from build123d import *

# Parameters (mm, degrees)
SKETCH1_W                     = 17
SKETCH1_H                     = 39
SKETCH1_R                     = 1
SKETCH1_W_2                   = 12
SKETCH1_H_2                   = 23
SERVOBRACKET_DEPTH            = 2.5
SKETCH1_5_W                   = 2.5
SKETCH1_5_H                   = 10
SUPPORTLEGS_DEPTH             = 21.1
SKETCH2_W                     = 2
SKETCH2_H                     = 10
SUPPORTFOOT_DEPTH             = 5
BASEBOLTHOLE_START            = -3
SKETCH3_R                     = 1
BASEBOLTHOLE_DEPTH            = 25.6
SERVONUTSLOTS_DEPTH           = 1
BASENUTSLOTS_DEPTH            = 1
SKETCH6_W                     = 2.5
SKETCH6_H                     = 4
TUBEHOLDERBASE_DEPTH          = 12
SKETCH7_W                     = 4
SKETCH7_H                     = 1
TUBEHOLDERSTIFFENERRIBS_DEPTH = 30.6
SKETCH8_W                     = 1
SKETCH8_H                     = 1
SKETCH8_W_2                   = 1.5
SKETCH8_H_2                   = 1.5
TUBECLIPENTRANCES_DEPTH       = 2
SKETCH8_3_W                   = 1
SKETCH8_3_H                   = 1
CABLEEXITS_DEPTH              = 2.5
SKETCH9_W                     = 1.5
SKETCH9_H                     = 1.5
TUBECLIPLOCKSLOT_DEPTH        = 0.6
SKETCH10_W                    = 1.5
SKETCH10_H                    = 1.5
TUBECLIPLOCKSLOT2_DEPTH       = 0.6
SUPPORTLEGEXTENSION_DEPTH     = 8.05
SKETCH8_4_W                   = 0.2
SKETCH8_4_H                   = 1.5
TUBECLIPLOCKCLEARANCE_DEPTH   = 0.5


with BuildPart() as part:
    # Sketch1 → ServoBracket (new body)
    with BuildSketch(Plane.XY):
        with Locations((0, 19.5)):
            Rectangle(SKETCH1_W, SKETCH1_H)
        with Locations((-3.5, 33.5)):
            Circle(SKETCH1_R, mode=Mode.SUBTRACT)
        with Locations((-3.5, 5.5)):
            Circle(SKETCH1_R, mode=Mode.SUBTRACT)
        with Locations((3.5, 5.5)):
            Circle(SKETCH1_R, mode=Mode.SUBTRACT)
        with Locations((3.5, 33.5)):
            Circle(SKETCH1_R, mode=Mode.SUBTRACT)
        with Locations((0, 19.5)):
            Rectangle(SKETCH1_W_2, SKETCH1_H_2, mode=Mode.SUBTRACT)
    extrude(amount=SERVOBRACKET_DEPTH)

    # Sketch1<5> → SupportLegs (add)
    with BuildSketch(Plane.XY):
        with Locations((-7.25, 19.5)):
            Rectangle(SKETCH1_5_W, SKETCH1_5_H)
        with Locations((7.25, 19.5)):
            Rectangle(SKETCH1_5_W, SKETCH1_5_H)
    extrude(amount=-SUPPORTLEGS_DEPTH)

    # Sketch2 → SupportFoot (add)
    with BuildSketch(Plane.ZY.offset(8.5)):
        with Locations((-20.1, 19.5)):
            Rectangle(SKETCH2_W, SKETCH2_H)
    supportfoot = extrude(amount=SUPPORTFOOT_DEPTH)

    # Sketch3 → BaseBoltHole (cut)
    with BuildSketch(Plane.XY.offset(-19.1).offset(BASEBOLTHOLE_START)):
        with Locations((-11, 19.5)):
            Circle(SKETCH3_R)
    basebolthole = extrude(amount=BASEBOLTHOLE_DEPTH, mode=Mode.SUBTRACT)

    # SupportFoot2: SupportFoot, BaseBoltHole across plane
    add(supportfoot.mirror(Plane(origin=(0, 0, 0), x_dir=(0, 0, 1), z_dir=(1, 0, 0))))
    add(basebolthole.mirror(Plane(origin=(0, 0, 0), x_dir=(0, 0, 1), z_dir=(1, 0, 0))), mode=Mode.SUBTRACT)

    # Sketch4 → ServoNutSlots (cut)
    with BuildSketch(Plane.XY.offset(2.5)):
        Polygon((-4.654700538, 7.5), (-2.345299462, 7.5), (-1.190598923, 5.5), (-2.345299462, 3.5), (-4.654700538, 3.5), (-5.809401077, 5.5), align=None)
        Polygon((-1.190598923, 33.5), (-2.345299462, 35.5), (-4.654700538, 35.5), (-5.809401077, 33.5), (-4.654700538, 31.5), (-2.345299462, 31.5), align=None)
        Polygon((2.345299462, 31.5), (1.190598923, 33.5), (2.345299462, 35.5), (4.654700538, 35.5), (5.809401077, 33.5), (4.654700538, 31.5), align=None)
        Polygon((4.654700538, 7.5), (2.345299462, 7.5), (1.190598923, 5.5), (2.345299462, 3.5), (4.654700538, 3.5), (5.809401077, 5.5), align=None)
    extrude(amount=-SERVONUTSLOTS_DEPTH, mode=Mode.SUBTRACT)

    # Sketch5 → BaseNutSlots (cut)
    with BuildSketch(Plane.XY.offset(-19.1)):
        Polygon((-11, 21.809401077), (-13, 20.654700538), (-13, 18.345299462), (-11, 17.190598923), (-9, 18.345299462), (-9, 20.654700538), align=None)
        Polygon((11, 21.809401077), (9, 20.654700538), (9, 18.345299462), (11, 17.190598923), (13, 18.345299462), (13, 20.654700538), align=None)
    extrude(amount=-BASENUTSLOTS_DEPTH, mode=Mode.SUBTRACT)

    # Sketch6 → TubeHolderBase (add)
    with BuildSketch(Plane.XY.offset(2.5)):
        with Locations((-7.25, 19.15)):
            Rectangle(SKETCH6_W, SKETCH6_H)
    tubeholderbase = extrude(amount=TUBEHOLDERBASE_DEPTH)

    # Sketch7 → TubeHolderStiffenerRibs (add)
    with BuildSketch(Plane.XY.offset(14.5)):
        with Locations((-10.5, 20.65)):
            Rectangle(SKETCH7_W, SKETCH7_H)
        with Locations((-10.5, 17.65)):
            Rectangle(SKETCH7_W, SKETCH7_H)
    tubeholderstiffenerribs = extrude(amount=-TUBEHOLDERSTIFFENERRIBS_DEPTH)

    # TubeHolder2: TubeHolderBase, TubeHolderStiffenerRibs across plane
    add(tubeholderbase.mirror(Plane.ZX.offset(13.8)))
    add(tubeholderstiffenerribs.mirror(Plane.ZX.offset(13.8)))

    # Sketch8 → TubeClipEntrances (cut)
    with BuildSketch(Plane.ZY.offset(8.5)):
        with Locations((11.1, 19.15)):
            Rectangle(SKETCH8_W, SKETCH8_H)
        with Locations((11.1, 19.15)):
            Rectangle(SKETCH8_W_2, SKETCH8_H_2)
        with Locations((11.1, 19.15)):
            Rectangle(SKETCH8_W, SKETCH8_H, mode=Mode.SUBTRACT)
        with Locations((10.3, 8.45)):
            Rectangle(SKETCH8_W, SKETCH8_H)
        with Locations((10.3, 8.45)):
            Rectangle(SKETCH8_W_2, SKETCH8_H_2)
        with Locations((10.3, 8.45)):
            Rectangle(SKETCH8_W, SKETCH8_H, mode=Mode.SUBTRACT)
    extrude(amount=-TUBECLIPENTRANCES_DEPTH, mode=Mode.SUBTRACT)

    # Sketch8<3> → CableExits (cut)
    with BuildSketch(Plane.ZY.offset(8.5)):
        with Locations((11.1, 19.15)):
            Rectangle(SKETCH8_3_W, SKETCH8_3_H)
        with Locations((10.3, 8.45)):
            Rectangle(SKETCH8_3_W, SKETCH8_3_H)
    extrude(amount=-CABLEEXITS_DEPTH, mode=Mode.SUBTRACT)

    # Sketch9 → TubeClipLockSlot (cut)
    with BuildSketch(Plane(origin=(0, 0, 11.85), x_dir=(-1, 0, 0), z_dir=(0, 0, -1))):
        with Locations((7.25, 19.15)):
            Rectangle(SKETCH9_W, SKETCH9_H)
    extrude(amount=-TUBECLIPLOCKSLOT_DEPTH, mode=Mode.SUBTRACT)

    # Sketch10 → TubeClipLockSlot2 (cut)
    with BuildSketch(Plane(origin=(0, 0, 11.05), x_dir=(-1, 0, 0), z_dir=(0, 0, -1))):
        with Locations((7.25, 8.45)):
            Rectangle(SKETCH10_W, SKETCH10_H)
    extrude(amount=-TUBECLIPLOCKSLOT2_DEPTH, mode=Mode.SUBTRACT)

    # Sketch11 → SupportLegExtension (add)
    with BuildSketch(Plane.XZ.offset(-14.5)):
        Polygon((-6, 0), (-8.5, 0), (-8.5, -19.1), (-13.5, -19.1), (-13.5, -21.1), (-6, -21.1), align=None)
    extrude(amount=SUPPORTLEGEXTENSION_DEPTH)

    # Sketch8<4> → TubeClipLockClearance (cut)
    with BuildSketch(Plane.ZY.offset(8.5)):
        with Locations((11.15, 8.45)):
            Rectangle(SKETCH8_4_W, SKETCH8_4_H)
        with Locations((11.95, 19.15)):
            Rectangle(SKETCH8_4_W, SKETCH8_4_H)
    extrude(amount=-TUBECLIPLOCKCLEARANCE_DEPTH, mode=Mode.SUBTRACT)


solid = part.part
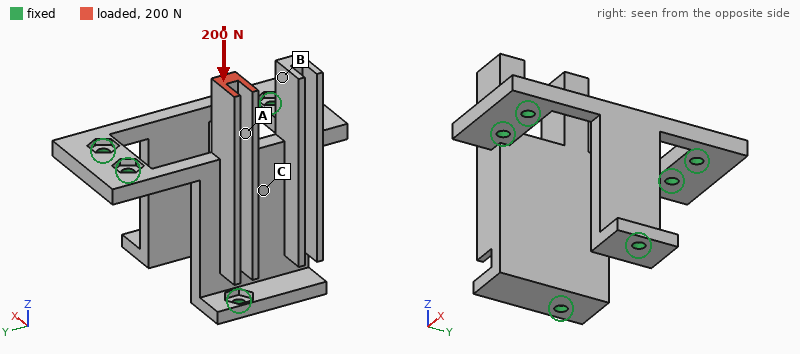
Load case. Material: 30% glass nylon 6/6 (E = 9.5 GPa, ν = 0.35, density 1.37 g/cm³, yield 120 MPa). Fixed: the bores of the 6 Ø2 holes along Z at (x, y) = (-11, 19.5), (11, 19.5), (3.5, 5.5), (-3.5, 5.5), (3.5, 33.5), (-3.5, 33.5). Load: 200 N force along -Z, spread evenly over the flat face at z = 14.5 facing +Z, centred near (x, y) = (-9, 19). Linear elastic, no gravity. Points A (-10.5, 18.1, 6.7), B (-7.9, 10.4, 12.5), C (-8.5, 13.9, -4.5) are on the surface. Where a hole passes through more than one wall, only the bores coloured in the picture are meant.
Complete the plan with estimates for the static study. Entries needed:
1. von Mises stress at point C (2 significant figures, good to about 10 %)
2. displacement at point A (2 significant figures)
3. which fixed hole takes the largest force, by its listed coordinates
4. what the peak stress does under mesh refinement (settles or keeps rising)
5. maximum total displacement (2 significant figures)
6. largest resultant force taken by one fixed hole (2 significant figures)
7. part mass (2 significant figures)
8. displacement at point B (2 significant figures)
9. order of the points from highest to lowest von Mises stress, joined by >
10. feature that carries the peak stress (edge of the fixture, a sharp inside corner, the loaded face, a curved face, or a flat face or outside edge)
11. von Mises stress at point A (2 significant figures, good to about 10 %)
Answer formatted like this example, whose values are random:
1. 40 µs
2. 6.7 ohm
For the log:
1. 7.1 MPa
2. 0.071 mm
3. (-11, 19.5)
4. keeps rising
5. 0.10 mm
6. 120 N
7. 4.6 g
8. 0.060 mm
9. A > C > B
10. edge of the fixture
11. 11 MPa
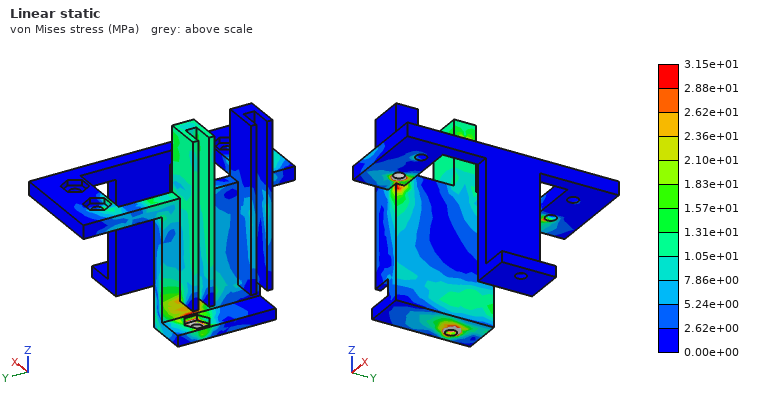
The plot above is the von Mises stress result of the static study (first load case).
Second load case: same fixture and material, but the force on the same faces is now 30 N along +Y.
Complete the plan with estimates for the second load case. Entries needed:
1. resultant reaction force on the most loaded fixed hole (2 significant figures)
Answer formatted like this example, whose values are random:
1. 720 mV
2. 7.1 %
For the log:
1. 27 N
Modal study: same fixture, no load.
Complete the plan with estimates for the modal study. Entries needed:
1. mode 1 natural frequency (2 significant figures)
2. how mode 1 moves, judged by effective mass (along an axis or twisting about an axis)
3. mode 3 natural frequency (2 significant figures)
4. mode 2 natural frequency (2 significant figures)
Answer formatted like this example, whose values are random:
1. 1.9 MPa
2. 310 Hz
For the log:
1. 3900 Hz
2. along X
3. 5300 Hz
4. 4800 Hz
